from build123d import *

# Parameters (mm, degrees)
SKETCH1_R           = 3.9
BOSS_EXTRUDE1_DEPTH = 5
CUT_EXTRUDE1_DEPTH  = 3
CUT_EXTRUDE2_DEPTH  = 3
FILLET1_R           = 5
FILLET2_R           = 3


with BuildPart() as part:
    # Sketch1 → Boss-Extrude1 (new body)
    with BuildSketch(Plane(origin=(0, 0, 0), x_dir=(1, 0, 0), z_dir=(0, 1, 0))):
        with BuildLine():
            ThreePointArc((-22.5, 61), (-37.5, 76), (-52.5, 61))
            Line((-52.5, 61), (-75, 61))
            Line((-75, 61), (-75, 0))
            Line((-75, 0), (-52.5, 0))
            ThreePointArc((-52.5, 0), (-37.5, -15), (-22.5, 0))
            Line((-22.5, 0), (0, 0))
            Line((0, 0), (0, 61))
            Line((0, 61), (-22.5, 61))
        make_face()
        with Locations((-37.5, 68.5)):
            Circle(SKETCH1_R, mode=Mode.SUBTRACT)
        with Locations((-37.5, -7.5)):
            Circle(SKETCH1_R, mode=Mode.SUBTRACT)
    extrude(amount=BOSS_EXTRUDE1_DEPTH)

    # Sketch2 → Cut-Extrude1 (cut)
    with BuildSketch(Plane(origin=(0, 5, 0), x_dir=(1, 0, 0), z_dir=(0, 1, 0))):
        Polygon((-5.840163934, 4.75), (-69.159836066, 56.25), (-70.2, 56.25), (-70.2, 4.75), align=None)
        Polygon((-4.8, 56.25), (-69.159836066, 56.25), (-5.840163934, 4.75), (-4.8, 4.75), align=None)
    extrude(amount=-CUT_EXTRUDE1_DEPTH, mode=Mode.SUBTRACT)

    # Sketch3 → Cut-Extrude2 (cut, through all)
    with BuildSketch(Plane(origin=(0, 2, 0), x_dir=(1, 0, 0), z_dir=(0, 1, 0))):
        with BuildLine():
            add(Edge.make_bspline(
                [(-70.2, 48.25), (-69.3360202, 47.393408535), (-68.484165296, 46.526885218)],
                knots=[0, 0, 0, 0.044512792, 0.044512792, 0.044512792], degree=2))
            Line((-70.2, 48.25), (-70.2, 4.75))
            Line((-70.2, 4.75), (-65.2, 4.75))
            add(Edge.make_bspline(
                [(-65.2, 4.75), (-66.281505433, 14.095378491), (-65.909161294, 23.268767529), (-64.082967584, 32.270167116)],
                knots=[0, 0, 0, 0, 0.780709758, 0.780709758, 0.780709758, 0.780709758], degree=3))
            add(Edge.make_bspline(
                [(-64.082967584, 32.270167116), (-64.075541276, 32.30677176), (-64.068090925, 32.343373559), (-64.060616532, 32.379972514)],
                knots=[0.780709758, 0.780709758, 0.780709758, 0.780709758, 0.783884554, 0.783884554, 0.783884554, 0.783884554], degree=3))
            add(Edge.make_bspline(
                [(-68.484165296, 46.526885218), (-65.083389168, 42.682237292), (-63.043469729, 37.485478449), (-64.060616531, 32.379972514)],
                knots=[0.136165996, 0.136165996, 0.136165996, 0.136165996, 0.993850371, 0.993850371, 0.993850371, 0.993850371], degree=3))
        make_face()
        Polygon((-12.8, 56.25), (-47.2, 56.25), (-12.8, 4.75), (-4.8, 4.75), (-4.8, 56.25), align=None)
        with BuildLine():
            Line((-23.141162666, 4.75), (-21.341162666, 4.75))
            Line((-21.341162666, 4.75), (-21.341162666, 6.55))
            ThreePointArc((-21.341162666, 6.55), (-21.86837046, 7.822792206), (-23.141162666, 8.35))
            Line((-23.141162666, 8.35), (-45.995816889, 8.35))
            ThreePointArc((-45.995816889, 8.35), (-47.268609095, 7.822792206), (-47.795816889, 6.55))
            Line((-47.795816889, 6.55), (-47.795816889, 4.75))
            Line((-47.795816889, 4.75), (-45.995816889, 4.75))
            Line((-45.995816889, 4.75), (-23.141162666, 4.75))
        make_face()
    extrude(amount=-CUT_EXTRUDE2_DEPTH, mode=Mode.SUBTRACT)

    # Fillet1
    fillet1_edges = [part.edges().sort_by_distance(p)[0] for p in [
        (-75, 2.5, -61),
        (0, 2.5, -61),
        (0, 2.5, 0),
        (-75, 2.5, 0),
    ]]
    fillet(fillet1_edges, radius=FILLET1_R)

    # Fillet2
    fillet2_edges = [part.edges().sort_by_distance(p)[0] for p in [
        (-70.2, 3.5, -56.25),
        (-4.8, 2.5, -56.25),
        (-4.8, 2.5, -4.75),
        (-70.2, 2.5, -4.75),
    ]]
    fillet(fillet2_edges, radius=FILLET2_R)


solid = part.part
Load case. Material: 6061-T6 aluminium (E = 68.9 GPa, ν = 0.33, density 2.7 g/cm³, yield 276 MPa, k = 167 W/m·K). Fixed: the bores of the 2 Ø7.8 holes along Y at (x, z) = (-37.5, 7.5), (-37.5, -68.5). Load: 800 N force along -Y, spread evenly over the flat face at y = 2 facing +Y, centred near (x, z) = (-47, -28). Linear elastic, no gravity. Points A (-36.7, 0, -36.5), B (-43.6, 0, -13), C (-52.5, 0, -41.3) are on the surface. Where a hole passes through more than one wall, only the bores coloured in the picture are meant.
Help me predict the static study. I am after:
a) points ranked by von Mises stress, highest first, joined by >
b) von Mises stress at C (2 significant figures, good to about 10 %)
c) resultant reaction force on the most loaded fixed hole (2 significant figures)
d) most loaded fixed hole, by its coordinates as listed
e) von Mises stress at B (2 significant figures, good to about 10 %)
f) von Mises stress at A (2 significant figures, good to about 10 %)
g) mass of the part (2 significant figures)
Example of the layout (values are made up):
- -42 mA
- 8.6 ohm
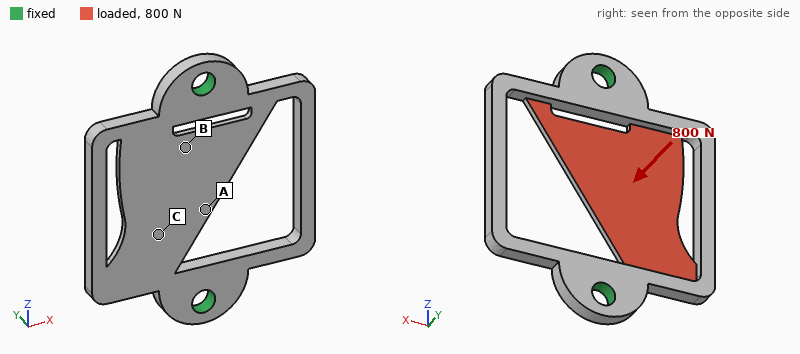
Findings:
- A > C > B
- 74 MPa
- 550 N
- (-37.5, 7.5)
- 26 MPa
- 120 MPa
- 34 g
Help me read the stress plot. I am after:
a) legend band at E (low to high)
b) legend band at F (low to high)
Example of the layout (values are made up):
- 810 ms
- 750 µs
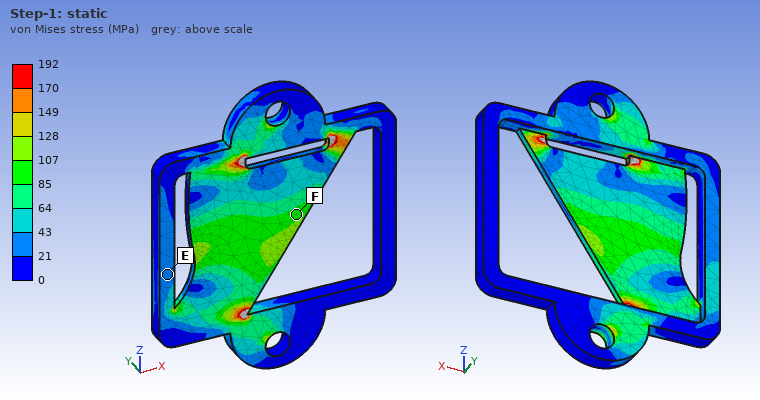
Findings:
- 21 to 43 MPa
- 85 to 107 MPa
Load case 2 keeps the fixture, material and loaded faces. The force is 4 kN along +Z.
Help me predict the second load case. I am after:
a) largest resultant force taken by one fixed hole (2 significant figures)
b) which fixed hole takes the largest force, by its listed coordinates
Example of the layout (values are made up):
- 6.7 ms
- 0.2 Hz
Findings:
- 2.3 kN
- (-37.5, 7.5)
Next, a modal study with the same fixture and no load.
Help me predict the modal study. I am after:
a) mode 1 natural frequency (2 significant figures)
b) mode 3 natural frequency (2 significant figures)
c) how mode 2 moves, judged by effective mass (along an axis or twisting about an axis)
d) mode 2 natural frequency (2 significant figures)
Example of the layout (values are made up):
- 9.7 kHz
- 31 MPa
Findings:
- 2000 Hz
- 2700 Hz
- along Y
- 2100 Hz
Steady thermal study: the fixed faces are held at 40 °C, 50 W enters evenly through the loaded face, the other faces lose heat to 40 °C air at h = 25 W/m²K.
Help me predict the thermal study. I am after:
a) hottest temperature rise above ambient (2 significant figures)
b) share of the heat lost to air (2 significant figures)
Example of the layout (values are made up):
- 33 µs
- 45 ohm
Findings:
- 74 K
- 12 %
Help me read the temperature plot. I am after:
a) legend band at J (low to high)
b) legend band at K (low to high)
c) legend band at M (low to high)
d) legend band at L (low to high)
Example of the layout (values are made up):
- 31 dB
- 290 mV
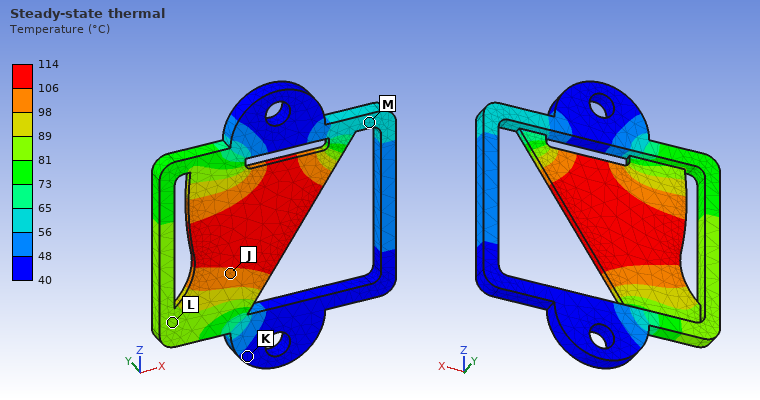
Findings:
- 98 to 106 °C
- 40 to 48 °C
- 56 to 65 °C
- 81 to 89 °C
